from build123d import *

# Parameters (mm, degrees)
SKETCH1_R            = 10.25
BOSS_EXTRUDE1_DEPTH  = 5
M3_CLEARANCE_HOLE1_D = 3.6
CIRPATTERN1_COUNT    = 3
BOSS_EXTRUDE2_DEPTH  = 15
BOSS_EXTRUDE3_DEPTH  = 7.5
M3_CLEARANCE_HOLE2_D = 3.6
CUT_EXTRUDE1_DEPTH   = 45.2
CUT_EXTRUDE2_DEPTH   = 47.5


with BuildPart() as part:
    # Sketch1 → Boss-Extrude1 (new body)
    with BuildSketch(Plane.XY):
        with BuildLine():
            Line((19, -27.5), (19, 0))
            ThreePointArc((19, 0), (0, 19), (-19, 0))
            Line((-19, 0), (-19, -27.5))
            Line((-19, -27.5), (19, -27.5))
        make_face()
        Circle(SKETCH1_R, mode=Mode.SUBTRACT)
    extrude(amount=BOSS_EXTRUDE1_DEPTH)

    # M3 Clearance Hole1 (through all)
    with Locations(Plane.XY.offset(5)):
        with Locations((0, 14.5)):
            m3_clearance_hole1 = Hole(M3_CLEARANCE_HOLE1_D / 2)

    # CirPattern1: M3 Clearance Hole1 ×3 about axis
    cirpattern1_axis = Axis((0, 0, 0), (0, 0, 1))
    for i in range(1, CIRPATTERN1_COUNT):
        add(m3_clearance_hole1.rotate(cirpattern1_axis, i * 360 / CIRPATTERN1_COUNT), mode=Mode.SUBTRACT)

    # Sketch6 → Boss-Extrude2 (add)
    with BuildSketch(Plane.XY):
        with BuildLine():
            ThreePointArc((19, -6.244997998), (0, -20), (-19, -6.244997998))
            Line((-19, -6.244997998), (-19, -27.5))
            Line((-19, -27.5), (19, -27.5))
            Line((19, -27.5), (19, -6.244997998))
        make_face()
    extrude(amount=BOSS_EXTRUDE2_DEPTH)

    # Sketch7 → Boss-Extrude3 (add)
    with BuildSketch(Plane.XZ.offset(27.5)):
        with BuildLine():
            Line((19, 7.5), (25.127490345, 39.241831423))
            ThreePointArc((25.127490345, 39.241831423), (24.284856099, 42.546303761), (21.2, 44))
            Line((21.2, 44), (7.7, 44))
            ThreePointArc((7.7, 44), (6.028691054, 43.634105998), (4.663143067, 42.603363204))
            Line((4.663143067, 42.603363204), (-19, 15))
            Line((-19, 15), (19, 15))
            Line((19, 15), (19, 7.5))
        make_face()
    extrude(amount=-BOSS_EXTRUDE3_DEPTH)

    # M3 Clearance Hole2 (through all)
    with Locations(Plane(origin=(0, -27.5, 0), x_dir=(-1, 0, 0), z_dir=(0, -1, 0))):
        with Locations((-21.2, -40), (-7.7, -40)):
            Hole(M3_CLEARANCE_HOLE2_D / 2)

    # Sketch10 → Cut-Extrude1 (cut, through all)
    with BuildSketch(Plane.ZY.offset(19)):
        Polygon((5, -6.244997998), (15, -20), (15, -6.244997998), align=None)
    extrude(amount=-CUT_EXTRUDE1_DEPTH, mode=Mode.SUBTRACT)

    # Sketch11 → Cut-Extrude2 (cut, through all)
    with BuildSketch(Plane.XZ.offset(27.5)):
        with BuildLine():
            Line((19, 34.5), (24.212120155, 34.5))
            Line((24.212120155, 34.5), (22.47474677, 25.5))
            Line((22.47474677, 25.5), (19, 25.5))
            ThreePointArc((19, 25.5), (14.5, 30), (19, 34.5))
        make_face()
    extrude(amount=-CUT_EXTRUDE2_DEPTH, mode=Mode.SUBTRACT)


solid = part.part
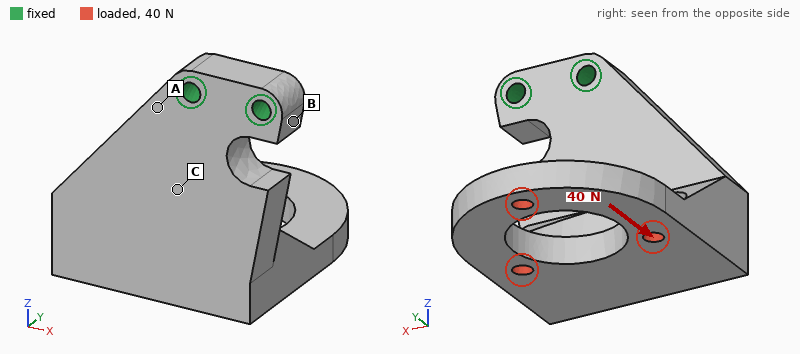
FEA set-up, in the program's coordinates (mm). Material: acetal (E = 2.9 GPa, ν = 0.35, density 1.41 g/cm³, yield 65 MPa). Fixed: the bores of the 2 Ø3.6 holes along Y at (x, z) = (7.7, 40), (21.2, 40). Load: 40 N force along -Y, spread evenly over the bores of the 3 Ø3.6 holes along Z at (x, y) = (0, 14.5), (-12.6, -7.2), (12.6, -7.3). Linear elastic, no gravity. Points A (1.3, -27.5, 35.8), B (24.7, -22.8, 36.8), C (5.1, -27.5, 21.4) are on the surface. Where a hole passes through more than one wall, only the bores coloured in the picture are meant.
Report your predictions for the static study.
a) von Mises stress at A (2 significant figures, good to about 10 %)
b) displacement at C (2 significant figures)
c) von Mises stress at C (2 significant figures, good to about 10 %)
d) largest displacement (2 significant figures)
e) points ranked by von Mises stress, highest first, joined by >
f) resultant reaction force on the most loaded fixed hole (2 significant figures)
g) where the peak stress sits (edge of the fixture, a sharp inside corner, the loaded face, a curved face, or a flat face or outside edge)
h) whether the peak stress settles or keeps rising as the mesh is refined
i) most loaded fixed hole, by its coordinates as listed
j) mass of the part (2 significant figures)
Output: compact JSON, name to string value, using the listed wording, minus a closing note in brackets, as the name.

{"von Mises stress at A": "7.1 MPa", "displacement at C": "0.15 mm", "von Mises stress at C": "3.0 MPa", "largest displacement": "0.75 mm", "points ranked by von Mises stress, highest first, joined by >": "A > C > B", "resultant reaction force on the most loaded fixed hole": "49 N", "where the peak stress sits": "edge of the fixture", "whether the peak stress settles or keeps rising as the mesh is refined": "keeps rising", "most loaded fixed hole, by its coordinates as listed": "(7.7, 40)", "mass of the part": "22 g"}
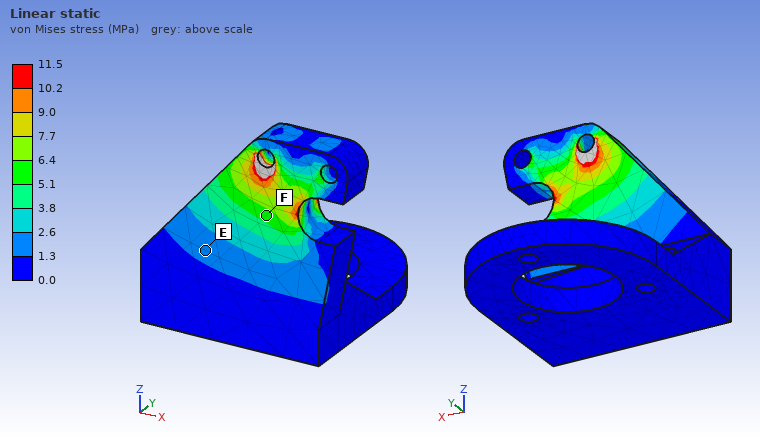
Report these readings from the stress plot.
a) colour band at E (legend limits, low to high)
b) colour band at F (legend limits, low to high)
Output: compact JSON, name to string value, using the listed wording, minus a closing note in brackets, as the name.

{"colour band at E": "1.3 to 2.6 MPa", "colour band at F": "5.1 to 6.4 MPa"}
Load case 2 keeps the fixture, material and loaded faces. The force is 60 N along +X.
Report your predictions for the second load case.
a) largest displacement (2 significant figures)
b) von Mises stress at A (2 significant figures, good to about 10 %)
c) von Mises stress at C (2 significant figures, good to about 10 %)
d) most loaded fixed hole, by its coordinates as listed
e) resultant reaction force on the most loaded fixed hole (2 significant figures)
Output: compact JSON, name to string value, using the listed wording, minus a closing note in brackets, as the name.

{"largest displacement": "0.84 mm", "von Mises stress at A": "9.9 MPa", "von Mises stress at C": "3.1 MPa", "most loaded fixed hole, by its coordinates as listed": "(21.2, 40)", "resultant reaction force on the most loaded fixed hole": "170 N"}
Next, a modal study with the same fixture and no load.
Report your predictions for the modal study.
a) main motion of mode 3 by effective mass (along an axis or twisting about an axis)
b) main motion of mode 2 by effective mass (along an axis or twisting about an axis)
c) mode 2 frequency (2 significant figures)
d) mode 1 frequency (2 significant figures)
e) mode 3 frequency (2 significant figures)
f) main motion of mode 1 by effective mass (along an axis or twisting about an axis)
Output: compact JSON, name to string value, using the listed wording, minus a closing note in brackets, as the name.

{"main motion of mode 3 by effective mass": "along X", "main motion of mode 2 by effective mass": "along X", "mode 2 frequency": "550 Hz", "mode 1 frequency": "370 Hz", "mode 3 frequency": "950 Hz", "main motion of mode 1 by effective mass": "along Y"}
